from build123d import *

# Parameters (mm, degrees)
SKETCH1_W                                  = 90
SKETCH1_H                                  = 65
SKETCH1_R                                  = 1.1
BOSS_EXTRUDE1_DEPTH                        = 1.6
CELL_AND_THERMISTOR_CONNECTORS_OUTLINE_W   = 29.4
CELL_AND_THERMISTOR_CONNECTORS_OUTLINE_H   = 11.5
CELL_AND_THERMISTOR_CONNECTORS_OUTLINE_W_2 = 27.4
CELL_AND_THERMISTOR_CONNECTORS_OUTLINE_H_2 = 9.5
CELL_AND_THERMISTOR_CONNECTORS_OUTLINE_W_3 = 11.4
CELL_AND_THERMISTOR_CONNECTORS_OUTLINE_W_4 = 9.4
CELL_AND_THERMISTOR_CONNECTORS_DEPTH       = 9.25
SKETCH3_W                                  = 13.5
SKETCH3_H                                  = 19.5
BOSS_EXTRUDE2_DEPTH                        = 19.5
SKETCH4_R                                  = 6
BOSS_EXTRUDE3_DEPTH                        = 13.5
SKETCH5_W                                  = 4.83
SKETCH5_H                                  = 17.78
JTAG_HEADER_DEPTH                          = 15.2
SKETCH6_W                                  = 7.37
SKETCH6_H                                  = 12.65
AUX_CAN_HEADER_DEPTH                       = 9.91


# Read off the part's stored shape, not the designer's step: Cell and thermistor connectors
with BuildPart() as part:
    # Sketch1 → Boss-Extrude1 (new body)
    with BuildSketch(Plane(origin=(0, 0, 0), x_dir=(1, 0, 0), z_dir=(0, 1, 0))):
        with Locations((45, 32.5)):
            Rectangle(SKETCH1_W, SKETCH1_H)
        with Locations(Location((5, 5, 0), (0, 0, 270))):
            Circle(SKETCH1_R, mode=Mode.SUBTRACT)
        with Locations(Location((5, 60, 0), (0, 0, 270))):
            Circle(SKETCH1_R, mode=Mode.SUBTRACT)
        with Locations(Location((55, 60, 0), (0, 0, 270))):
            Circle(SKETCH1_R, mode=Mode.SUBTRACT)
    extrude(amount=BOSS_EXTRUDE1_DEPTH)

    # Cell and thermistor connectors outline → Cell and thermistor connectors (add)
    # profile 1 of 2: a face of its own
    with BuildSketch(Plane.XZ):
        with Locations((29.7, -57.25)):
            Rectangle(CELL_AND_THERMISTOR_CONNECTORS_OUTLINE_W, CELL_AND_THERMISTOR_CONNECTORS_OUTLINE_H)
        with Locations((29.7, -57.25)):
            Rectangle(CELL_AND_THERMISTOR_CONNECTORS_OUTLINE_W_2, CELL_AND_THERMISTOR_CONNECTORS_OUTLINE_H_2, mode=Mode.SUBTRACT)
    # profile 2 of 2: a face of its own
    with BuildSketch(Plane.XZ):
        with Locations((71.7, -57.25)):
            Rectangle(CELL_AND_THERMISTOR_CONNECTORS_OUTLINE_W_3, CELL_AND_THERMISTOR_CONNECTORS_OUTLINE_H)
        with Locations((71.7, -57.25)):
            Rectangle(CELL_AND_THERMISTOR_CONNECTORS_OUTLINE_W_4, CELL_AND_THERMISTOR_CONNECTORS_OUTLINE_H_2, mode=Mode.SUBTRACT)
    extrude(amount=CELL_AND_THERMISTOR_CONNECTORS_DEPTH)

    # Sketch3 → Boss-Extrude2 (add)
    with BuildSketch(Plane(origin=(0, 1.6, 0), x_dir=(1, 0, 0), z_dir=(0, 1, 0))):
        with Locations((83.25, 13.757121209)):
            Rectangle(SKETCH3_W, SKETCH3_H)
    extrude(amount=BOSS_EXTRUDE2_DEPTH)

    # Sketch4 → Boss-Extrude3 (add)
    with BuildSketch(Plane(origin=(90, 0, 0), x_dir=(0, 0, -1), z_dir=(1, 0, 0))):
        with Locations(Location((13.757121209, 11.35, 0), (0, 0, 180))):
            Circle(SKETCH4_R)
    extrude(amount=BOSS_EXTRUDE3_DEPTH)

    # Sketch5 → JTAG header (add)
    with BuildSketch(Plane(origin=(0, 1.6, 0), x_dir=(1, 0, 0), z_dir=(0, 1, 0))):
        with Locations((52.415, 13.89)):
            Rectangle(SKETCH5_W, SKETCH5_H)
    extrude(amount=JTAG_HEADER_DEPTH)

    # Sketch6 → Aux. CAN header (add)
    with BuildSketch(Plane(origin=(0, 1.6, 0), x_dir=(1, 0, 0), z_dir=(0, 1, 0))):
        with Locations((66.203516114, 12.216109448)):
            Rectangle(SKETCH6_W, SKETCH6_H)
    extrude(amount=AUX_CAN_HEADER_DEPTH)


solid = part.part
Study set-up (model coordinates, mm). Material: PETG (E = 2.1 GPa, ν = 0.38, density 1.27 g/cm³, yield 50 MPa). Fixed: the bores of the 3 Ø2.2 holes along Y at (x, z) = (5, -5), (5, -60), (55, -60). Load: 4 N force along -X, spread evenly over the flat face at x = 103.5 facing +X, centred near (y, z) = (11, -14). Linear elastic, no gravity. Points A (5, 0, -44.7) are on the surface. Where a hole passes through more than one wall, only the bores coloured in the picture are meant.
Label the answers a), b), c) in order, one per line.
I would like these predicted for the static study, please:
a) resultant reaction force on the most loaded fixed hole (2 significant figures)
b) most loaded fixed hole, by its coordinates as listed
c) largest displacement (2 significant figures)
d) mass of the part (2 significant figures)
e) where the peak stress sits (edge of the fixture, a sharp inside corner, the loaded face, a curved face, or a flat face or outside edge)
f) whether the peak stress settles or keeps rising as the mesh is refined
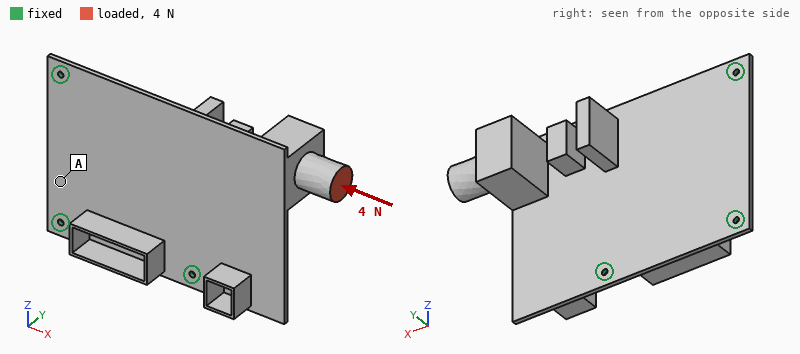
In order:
a) 2.6 N
b) (5, -5)
c) 1.4 mm
d) 25 g
e) edge of the fixture
f) keeps rising
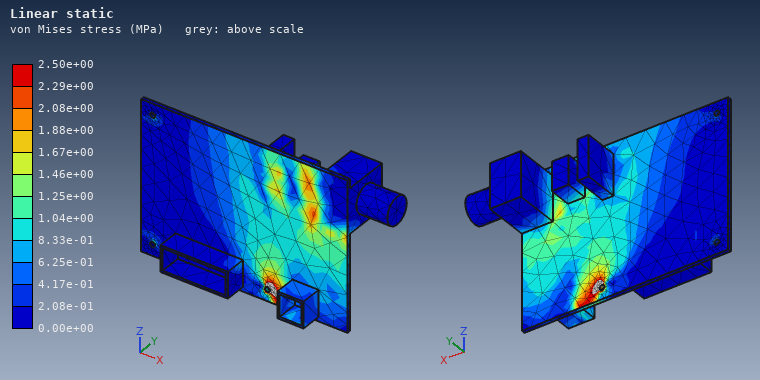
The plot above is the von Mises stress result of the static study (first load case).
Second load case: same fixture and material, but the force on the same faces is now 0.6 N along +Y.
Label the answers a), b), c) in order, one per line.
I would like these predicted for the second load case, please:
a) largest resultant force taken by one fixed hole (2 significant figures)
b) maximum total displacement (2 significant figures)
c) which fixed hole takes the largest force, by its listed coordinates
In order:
a) 0.88 N
b) 1.3 mm
c) (55, -60)
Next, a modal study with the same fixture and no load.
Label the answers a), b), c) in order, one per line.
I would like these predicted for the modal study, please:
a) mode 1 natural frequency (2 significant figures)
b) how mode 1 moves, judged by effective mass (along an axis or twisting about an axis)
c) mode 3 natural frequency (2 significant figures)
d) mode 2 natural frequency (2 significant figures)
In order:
a) 44 Hz
b) along Y
c) 260 Hz
d) 150 Hz
